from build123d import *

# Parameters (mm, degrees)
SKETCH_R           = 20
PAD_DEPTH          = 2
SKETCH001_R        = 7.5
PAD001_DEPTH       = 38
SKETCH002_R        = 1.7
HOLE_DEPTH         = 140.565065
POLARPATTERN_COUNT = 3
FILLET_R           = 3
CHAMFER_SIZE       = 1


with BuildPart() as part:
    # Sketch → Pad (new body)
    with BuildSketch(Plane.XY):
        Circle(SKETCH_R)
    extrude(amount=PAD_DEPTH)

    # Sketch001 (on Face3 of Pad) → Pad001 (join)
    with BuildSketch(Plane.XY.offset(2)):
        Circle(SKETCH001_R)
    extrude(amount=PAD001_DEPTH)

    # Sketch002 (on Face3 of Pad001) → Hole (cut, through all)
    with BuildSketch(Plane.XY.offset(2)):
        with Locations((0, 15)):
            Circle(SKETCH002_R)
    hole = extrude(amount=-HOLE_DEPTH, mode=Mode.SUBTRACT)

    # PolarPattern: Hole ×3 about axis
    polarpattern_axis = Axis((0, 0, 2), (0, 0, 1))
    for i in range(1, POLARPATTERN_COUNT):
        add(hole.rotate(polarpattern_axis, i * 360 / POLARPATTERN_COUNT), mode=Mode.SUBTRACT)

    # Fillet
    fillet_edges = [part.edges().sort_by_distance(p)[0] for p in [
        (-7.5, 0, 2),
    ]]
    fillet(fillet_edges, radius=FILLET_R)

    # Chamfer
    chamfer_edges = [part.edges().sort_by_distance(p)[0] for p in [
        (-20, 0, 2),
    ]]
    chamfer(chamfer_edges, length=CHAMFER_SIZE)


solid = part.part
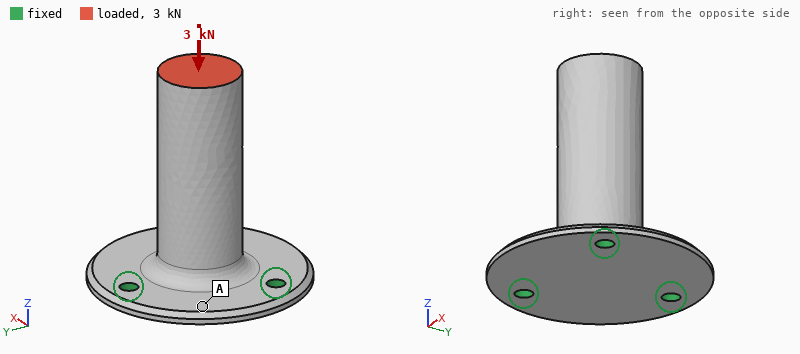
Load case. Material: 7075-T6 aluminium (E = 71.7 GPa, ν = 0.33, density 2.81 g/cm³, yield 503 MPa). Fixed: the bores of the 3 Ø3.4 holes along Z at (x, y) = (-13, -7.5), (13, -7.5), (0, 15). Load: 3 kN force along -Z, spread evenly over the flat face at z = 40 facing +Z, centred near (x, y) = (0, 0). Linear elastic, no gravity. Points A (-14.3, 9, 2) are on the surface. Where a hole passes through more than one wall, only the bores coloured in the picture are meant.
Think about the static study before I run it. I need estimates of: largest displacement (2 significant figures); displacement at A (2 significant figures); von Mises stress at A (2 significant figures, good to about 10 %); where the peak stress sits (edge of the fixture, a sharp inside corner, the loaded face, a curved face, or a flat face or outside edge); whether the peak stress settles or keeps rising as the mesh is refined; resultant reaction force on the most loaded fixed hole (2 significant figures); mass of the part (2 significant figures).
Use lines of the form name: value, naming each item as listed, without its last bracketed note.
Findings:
largest displacement: 62 µm
displacement at A: 40 µm
von Mises stress at A: 50 MPa
where the peak stress sits: edge of the fixture
whether the peak stress settles or keeps rising as the mesh is refined: keeps rising
resultant reaction force on the most loaded fixed hole: 1.1 kN
mass of the part: 26 g
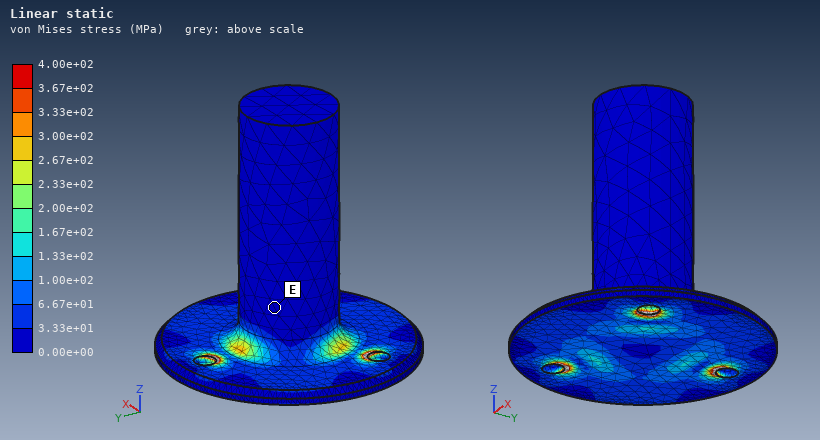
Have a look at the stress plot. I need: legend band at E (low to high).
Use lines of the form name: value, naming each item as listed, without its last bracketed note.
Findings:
legend band at E: 0.00e+00 to 3.33e+01 MPa
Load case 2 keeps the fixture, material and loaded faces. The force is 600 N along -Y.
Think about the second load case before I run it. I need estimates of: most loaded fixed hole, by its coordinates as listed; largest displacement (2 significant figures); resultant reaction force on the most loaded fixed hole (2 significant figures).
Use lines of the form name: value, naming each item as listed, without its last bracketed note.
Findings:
most loaded fixed hole, by its coordinates as listed: (0, 15)
largest displacement: 0.29 mm
resultant reaction force on the most loaded fixed hole: 1.3 kN
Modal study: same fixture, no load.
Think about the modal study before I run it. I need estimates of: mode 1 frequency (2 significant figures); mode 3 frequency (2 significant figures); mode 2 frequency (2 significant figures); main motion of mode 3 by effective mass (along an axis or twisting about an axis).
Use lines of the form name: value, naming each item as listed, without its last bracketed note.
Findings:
mode 1 frequency: 2900 Hz
mode 3 frequency: 7800 Hz
mode 2 frequency: 2900 Hz
main motion of mode 3 by effective mass: along Z
